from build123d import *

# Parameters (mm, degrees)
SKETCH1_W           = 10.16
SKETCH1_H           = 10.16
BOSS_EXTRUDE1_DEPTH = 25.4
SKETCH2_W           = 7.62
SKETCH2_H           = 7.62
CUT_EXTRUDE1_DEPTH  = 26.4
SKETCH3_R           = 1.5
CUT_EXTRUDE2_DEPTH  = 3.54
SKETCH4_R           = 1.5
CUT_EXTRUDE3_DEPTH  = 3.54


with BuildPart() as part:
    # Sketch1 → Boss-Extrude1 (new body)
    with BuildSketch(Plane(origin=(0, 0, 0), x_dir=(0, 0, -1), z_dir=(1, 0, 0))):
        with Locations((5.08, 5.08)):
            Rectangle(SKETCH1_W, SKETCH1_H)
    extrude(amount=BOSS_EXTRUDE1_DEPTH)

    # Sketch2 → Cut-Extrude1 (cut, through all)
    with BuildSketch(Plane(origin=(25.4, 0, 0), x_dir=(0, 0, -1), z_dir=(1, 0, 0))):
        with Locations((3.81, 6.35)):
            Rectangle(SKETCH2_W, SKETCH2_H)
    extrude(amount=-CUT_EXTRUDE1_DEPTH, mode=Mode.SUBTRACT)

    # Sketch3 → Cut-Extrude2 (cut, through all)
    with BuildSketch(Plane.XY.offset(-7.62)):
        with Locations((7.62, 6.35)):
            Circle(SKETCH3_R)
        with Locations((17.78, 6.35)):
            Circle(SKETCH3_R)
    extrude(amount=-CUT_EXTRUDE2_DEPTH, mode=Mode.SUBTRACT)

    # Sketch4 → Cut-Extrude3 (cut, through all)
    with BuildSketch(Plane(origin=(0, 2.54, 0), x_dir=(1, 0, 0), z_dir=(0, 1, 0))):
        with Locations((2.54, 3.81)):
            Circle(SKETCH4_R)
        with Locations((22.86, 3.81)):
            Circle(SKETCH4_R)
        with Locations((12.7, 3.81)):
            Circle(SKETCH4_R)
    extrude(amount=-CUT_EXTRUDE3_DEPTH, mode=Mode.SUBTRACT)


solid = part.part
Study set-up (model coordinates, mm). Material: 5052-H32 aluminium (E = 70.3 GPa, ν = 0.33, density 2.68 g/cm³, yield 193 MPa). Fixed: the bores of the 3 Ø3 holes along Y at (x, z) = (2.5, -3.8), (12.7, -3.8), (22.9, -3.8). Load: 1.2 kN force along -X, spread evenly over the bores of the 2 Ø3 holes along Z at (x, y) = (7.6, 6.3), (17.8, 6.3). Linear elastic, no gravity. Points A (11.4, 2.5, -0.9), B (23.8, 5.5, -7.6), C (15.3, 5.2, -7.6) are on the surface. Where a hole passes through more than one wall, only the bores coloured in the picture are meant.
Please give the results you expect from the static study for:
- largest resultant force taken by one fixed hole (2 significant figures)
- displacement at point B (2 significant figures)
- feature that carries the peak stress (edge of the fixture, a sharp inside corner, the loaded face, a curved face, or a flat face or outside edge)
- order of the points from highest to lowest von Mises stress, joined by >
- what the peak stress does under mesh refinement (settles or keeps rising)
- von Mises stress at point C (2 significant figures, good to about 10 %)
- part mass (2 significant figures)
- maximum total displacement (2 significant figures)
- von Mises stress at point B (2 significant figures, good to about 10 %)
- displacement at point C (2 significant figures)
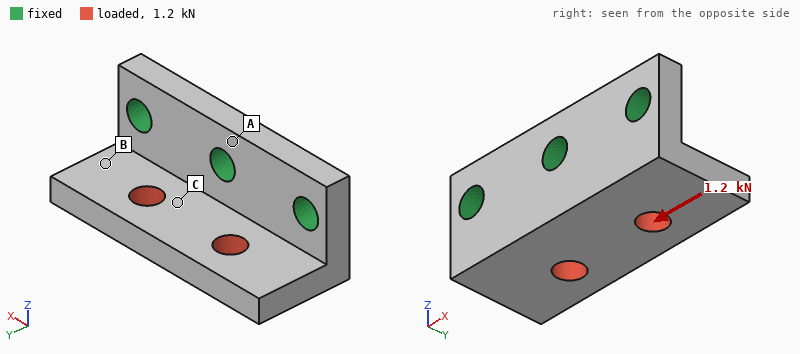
520 N
15 µm
edge of the fixture
C > B > A
keeps rising
55 MPa
2.8 g
26 µm
32 MPa
10 µm
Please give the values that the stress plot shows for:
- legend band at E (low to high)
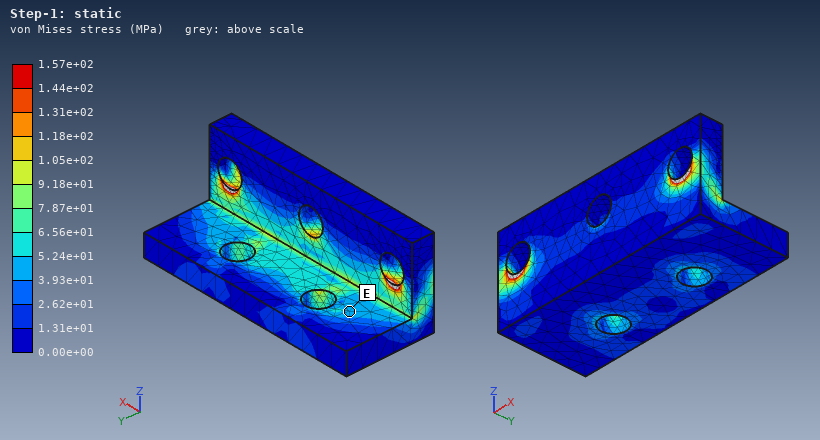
3.93e+01 to 5.24e+01 MPa
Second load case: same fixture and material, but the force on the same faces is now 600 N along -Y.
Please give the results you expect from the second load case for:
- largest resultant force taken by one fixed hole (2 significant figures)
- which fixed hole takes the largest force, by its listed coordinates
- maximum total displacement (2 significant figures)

260 N
(12.7, -3.8)
26 µm
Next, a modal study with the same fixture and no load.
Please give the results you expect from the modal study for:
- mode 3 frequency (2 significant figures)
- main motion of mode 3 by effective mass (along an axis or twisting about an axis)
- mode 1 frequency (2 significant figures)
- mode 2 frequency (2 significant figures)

41 kHz
along X
16 kHz
22 kHz
